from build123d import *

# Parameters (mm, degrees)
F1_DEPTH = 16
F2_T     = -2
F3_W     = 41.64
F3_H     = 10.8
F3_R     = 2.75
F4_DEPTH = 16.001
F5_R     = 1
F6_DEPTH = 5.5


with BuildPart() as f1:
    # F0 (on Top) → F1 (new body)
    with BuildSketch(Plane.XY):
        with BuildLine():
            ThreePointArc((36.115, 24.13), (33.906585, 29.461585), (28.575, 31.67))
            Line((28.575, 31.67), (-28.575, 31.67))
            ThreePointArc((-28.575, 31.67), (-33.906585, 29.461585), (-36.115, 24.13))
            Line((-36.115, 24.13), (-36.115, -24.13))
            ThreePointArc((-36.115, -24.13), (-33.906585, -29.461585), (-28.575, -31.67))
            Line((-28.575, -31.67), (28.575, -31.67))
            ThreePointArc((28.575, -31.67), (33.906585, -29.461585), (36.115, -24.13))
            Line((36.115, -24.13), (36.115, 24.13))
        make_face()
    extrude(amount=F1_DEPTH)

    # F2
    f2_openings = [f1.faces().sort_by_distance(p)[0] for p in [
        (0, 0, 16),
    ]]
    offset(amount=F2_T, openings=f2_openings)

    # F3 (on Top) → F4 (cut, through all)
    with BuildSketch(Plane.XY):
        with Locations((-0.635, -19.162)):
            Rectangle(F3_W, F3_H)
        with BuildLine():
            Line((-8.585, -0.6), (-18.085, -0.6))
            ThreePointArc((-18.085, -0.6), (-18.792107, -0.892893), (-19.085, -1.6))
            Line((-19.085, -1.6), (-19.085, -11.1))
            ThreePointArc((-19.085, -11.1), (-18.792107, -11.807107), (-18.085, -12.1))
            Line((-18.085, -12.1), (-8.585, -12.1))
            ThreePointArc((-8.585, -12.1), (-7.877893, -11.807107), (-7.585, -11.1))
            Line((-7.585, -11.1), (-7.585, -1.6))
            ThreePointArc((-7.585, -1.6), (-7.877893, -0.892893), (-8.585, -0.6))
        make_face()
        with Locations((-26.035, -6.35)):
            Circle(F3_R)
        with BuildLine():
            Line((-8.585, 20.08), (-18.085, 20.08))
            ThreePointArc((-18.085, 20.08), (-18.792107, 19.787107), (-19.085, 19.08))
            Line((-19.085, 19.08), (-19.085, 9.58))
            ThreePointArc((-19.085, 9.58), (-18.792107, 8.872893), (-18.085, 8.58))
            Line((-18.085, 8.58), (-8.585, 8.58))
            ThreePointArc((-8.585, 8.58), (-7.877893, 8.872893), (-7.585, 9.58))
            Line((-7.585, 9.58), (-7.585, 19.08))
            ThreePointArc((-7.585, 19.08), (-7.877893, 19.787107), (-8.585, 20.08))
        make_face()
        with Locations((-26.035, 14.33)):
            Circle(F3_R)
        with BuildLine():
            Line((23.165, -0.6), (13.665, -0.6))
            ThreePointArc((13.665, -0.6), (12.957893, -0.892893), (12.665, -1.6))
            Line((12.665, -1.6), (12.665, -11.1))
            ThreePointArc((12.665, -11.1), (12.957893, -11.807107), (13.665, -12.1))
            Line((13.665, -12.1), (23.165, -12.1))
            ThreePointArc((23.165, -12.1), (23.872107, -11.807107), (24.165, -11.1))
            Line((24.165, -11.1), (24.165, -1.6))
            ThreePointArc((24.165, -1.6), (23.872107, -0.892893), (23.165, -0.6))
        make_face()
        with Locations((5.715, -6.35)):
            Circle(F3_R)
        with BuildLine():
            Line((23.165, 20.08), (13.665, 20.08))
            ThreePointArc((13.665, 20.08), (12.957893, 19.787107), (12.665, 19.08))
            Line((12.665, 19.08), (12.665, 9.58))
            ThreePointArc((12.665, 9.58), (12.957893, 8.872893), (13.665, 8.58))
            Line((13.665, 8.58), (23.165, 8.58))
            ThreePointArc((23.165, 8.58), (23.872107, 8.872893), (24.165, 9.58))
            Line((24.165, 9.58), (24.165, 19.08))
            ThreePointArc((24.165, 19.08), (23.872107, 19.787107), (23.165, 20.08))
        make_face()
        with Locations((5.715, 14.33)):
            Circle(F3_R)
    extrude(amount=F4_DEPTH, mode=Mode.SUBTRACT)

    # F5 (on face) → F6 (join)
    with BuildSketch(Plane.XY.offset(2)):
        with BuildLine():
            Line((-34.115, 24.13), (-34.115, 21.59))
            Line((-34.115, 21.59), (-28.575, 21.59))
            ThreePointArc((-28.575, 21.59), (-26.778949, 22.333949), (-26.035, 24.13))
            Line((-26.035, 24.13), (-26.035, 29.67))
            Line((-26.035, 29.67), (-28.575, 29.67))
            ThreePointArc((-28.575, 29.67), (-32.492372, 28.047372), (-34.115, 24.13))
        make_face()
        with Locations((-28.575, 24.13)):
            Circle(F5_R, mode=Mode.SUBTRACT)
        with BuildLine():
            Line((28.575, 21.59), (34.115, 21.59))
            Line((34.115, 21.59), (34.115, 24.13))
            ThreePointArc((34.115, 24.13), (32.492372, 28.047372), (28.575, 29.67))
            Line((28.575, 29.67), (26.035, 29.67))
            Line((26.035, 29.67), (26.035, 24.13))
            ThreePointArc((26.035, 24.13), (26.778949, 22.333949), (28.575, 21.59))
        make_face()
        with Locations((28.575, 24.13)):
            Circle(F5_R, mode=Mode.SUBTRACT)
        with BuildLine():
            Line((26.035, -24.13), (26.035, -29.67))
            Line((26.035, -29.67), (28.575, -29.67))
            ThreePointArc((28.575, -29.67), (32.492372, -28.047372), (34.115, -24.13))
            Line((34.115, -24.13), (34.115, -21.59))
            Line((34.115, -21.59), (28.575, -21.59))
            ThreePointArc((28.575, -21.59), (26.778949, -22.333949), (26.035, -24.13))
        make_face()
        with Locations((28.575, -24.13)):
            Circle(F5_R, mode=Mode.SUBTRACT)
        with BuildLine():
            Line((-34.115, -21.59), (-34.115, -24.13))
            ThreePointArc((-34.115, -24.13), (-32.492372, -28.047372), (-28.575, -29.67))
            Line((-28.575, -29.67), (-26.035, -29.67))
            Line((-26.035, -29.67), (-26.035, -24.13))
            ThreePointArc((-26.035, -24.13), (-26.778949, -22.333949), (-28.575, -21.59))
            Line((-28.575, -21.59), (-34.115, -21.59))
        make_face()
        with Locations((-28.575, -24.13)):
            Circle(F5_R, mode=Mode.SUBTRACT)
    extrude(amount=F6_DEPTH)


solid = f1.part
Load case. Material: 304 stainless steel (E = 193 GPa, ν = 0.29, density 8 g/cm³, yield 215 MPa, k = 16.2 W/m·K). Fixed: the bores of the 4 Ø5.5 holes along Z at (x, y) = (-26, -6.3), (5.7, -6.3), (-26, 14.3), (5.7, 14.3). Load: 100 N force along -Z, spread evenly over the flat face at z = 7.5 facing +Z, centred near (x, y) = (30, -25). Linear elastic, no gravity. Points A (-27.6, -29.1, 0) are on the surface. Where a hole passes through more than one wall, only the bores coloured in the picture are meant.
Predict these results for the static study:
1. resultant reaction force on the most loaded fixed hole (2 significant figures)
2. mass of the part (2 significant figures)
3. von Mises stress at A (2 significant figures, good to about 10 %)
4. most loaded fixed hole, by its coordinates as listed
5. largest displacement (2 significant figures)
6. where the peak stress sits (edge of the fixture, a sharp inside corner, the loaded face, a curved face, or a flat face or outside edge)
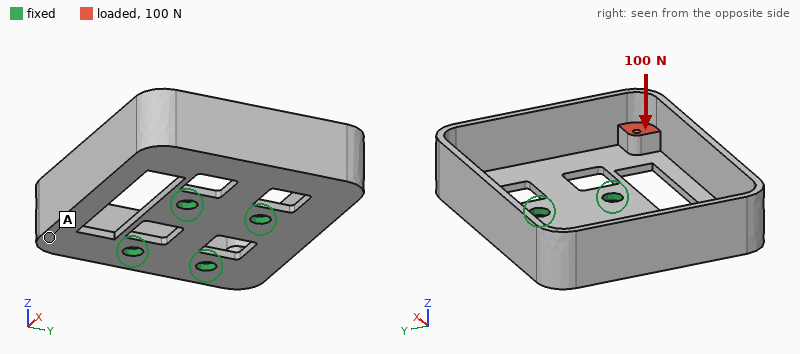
99 N
120 g
15 MPa
(5.7, -6.3)
0.19 mm
a curved face
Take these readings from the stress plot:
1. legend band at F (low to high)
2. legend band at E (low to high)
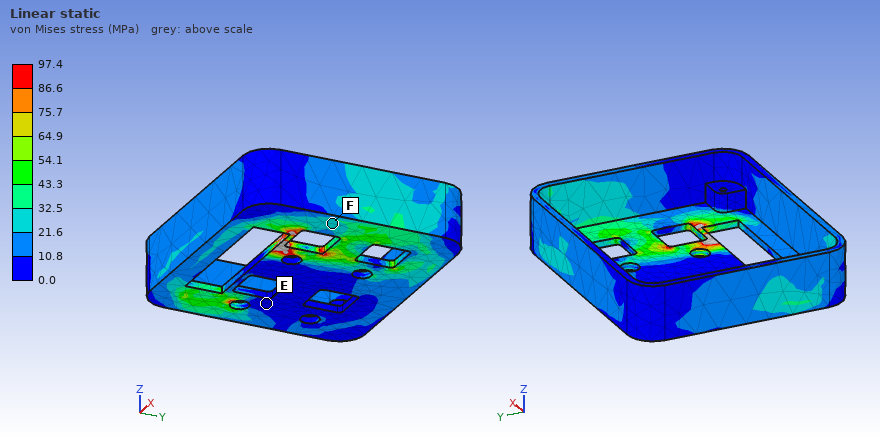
21.6 to 32.5 MPa
0.0 to 10.8 MPa
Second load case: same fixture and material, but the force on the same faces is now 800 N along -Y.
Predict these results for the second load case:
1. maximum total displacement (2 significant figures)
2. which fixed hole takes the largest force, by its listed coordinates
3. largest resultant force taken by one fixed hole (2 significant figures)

0.23 mm
(5.7, 14.3)
770 N
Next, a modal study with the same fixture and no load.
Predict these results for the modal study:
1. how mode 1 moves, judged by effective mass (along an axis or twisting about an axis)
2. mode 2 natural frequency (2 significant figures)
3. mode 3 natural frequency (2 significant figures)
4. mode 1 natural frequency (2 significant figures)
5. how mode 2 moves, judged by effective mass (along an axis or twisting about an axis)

along Z
1700 Hz
3100 Hz
860 Hz
along Z
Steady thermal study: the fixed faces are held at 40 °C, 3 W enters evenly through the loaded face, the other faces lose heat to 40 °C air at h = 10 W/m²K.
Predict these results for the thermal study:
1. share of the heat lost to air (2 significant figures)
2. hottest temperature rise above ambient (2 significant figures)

69 %
72 K
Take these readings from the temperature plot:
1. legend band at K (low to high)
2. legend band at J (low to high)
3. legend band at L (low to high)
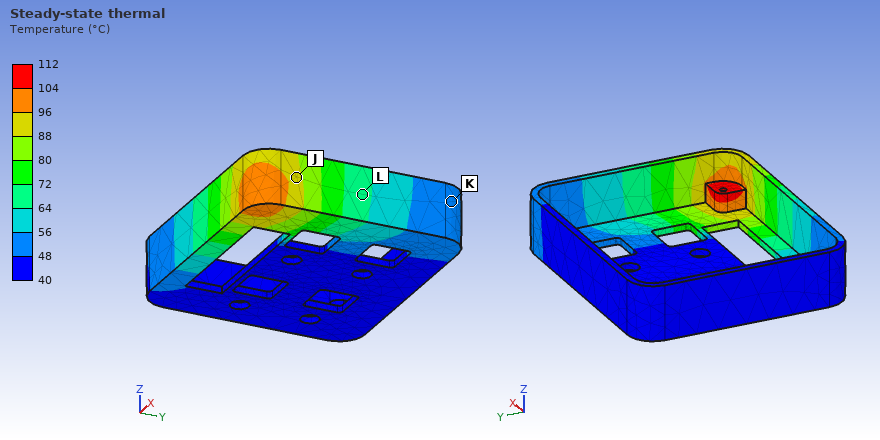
48 to 56 °C
88 to 96 °C
64 to 72 °C
